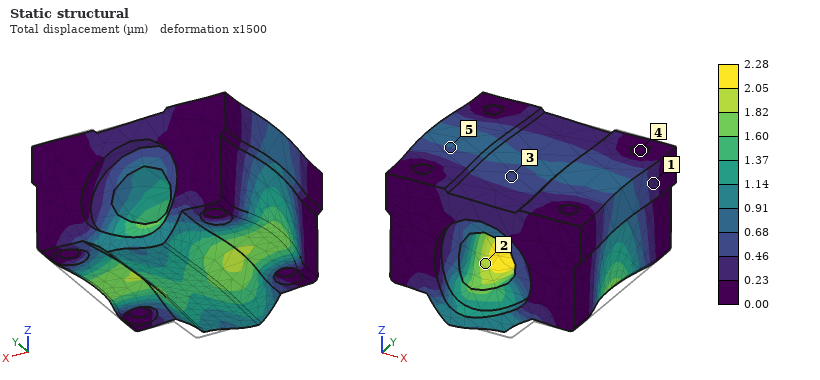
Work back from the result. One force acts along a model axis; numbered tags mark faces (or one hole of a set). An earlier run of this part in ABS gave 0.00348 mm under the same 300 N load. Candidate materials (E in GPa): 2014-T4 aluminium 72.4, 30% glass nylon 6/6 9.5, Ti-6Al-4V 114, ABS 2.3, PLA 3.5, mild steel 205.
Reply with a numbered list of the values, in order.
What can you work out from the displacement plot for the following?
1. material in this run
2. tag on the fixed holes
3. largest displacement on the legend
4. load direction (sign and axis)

1. PLA
2. 4
3. 2.28 µm
4. -X
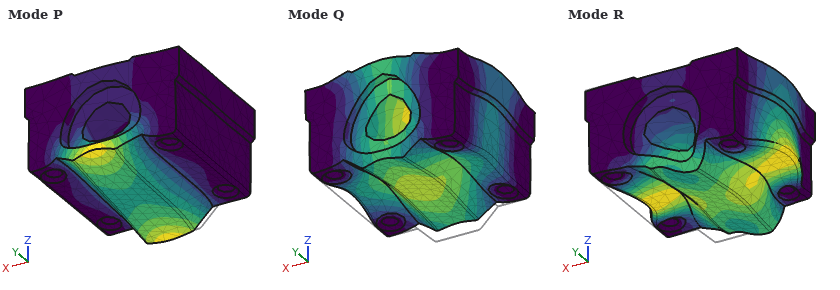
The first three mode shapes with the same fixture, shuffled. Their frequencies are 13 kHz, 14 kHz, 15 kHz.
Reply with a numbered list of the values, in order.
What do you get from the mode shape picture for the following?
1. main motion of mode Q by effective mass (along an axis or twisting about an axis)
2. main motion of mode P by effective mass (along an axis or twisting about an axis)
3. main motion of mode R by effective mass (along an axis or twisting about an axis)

1. along Z
2. along Y
3. along X
